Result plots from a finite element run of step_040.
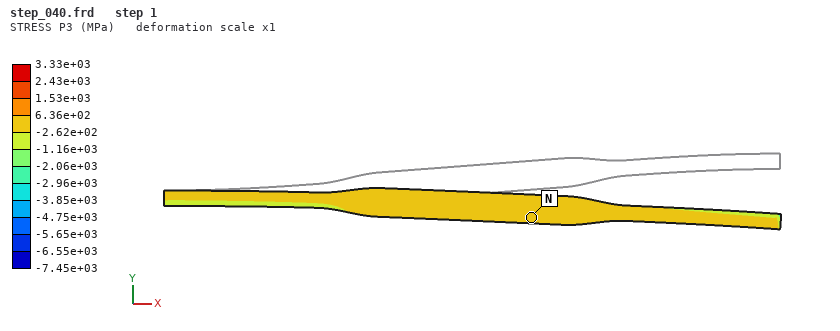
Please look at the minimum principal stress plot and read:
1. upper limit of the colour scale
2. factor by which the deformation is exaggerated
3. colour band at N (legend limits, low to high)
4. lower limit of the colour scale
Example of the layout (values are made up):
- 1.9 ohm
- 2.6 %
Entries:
- 3.33e+03 MPa
- 1
- -2.62e+02 to 6.36e+02 MPa
- -7.45e+03 MPa
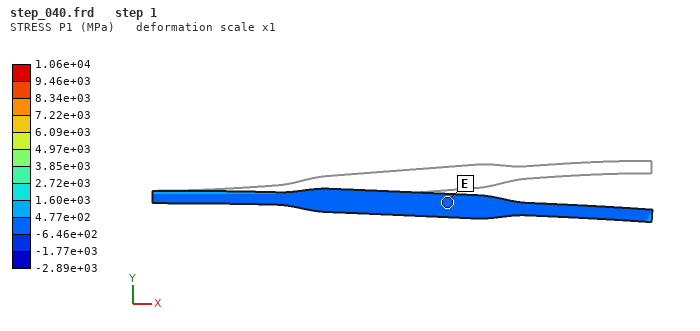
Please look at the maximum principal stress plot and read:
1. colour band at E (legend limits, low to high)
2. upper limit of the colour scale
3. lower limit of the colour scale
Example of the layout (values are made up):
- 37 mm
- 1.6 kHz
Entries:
- -6.46e+02 to 4.77e+02 MPa
- 1.06e+04 MPa
- -2.89e+03 MPa
